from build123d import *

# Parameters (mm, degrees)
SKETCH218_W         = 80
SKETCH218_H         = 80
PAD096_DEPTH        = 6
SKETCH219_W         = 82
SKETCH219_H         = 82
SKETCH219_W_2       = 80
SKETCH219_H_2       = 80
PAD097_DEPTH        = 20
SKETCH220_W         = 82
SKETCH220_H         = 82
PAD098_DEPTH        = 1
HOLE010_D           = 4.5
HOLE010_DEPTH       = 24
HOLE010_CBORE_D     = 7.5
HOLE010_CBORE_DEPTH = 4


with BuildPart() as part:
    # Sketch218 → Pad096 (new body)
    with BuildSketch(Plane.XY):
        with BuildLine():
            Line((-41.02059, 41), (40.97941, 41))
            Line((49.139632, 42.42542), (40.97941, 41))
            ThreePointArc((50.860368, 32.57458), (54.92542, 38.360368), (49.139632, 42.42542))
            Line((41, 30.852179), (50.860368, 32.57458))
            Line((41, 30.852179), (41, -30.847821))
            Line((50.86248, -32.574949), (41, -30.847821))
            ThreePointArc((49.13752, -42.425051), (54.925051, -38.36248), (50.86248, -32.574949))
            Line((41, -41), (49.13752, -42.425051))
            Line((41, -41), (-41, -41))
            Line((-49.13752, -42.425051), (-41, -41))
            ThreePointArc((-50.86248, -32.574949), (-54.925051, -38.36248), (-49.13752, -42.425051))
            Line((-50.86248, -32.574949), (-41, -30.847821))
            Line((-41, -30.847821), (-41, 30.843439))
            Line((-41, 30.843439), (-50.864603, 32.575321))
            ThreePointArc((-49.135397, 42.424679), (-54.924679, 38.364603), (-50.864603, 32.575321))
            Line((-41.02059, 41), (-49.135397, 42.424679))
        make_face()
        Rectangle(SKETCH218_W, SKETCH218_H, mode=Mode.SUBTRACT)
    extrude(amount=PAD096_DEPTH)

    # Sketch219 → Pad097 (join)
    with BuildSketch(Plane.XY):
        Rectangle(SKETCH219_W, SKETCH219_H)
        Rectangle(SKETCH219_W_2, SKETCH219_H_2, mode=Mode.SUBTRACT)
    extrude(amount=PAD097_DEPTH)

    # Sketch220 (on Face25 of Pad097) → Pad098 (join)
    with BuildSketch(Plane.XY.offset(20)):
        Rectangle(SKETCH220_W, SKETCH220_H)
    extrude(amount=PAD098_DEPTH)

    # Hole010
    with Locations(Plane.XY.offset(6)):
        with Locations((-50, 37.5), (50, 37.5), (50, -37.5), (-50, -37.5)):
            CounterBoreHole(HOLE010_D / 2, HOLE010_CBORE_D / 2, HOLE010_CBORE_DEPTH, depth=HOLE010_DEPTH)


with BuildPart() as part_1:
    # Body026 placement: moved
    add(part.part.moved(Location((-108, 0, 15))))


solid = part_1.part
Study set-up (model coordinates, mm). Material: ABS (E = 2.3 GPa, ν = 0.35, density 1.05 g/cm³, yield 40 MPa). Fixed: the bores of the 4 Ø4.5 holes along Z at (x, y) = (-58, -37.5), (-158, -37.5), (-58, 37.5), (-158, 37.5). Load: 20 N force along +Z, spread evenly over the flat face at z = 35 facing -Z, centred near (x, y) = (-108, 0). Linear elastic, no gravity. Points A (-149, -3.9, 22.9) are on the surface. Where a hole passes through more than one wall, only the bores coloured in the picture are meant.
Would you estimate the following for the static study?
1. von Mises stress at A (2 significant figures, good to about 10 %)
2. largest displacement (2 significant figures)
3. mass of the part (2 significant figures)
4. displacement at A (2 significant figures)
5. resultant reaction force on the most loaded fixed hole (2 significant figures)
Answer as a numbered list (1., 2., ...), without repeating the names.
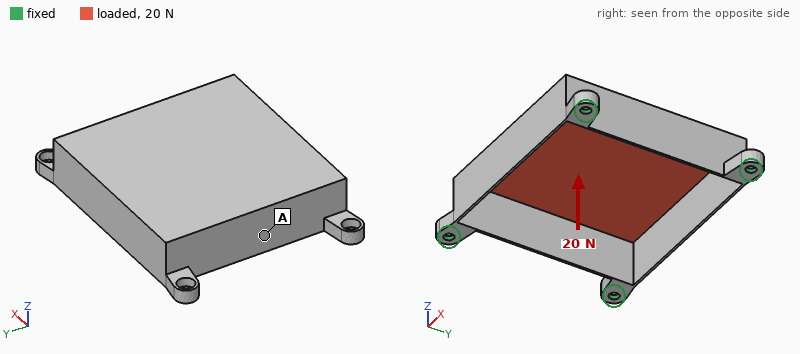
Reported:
1. 1.5 MPa
2. 1.4 mm
3. 16 g
4. 0.29 mm
5. 7.0 N
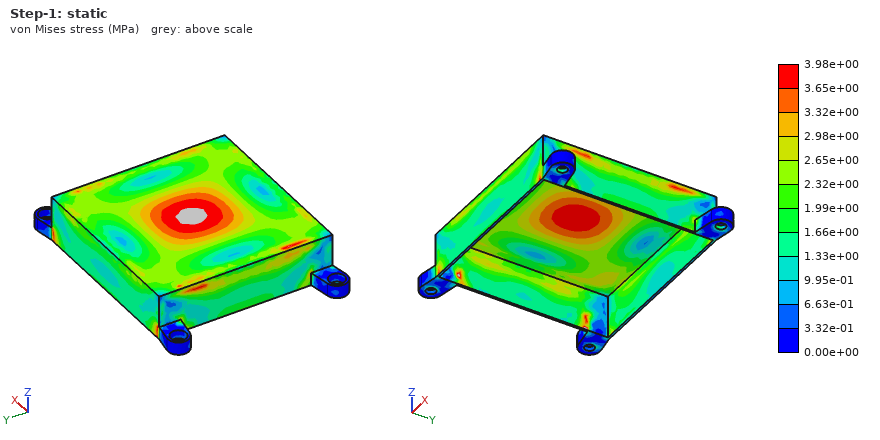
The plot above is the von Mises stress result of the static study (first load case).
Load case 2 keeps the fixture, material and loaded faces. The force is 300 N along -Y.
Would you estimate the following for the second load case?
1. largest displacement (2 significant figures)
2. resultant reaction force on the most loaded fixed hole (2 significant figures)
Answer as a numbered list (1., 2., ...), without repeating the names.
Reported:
1. 0.25 mm
2. 82 N
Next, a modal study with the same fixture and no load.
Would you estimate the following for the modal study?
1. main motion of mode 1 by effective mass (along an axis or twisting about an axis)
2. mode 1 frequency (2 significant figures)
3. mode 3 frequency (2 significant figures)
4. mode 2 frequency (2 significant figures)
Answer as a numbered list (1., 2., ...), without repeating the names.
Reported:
1. along Z
2. 280 Hz
3. 570 Hz
4. 480 Hz
